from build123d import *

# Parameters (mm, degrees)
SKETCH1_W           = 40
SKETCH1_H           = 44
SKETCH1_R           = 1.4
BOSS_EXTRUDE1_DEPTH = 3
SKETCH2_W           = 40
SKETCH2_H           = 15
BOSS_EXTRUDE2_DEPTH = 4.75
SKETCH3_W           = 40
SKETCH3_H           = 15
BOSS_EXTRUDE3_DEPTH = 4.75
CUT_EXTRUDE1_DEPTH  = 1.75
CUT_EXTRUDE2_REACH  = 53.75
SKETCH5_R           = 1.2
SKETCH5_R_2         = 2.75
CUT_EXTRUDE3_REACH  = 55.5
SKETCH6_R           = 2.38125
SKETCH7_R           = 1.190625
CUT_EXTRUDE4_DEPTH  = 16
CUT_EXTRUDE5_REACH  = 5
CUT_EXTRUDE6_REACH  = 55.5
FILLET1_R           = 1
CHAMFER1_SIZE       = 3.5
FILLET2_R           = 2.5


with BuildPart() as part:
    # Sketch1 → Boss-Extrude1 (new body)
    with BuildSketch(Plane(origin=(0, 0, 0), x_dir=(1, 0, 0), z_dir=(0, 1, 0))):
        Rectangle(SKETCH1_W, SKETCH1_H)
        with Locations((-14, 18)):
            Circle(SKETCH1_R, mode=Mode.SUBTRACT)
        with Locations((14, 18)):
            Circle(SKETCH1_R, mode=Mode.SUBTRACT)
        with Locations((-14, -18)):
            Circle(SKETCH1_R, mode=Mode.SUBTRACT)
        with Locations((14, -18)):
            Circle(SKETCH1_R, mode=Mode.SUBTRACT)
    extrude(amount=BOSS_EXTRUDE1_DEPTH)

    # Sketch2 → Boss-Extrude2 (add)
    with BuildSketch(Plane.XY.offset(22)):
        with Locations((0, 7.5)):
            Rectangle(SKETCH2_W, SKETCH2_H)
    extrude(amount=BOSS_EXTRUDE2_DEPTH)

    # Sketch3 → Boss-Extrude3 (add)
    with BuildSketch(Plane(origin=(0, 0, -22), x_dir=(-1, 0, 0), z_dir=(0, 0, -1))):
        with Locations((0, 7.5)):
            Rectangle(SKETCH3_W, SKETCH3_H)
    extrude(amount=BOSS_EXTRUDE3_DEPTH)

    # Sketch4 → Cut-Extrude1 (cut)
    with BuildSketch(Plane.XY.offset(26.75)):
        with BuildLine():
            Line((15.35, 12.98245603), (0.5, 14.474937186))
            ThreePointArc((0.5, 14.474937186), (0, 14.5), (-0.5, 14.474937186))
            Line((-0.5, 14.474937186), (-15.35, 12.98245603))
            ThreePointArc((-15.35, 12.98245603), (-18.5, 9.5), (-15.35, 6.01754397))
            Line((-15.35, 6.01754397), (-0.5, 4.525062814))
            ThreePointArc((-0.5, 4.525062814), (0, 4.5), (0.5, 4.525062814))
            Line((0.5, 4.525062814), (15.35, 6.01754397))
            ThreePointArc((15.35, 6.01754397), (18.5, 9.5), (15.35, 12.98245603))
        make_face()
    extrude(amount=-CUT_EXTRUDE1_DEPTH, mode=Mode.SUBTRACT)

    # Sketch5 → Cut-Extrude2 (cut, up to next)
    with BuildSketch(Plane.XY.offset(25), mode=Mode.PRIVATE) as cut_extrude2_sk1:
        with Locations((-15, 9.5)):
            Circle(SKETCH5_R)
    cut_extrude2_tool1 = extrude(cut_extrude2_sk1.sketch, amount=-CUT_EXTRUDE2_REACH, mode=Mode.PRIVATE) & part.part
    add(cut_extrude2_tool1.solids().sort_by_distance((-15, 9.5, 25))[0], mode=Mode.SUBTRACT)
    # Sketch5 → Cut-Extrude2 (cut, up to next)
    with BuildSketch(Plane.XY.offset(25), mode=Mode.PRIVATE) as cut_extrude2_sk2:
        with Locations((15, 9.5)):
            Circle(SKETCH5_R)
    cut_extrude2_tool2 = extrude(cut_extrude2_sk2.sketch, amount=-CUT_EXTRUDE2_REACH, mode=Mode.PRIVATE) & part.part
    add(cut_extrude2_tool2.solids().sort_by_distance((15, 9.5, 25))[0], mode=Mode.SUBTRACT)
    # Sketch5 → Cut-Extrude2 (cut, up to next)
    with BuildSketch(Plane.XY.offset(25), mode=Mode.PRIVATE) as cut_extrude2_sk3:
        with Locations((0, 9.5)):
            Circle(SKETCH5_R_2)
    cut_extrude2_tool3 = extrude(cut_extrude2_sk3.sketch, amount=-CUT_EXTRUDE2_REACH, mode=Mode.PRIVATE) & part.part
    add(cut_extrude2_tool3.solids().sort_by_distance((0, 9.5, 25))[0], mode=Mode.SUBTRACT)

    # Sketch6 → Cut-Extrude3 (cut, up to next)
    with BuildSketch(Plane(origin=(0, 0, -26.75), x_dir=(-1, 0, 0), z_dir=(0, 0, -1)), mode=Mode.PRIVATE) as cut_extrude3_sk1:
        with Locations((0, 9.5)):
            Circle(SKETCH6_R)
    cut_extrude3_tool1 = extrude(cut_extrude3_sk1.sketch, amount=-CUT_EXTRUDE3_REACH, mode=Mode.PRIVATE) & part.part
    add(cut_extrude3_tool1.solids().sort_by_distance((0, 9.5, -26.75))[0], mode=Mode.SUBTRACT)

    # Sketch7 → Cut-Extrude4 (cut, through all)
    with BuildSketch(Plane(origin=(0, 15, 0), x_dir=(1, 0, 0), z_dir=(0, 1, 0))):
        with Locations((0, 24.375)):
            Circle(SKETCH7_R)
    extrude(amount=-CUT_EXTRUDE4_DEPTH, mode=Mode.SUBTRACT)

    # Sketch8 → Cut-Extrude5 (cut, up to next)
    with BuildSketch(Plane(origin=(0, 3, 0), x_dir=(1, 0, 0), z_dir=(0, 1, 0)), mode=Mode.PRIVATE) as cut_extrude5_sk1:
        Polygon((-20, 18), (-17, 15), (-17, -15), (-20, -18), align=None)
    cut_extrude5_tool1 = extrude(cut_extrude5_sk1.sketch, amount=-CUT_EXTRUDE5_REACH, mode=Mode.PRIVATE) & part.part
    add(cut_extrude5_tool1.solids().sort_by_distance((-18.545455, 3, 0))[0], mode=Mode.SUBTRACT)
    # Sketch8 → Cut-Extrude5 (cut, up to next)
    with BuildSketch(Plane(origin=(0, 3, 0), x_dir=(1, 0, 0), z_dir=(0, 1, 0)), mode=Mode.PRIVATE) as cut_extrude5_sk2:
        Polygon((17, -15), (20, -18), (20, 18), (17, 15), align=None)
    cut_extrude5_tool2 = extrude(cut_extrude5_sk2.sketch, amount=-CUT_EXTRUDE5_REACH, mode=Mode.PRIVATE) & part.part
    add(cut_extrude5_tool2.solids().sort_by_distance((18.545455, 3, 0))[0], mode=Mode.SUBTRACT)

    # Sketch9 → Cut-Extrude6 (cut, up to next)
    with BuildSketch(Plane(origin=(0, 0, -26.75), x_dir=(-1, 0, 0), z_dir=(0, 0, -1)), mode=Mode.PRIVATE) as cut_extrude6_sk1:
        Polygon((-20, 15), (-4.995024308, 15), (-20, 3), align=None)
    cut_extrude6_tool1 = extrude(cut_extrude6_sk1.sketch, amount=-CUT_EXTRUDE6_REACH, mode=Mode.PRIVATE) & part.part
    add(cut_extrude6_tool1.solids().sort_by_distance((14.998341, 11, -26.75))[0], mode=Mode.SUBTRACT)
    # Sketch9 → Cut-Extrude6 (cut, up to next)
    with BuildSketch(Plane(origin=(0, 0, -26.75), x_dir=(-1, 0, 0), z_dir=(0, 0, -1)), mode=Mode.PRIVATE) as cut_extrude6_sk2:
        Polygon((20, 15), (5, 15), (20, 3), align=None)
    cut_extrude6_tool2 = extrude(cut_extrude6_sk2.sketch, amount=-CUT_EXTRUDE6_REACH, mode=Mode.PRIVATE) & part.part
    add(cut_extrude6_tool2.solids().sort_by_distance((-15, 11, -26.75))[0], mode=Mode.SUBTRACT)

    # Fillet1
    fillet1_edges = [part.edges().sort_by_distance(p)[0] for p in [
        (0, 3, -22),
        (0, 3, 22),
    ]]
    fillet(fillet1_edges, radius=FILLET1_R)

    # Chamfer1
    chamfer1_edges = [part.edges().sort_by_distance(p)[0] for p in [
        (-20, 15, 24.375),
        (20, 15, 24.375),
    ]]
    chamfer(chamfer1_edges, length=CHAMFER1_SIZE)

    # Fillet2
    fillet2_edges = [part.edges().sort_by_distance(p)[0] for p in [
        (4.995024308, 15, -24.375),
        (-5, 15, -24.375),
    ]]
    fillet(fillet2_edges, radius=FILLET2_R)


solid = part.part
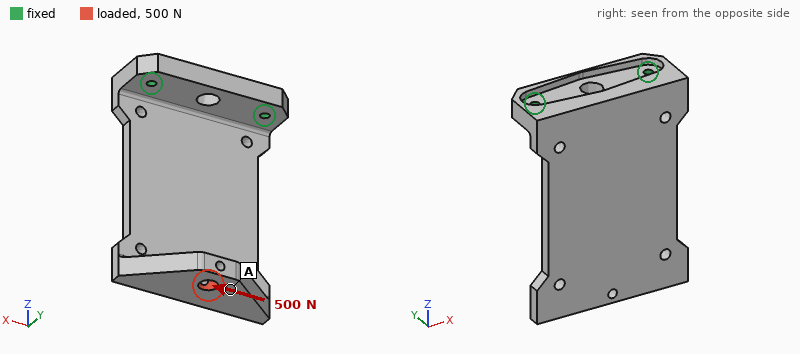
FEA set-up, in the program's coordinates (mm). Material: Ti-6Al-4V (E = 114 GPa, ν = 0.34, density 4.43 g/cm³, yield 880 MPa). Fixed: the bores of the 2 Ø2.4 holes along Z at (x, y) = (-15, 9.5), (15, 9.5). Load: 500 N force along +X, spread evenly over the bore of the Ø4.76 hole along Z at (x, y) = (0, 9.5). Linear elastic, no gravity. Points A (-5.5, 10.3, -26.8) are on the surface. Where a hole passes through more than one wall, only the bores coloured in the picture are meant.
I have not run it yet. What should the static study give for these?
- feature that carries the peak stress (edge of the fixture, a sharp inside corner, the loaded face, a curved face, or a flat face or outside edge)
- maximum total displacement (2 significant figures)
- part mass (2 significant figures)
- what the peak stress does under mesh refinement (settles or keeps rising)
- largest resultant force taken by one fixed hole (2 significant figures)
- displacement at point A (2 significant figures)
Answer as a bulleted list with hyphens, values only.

- edge of the fixture
- 0.29 mm
- 38 g
- keeps rising
- 800 N
- 0.24 mm
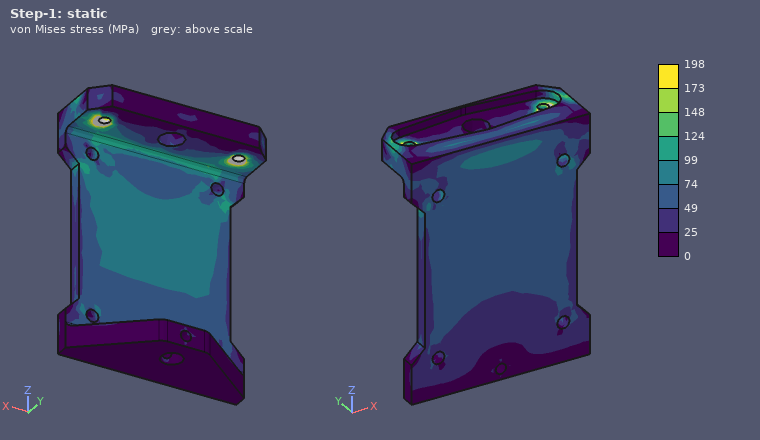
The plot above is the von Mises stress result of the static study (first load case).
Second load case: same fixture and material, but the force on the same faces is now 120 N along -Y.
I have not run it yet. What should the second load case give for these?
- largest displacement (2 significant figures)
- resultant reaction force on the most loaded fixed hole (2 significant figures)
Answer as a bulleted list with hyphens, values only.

- 0.72 mm
- 61 N
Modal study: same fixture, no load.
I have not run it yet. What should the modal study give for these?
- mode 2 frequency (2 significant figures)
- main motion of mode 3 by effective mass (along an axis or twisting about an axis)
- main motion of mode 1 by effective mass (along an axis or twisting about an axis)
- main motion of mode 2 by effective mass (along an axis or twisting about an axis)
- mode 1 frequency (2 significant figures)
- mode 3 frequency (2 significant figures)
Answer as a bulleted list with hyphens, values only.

- 2100 Hz
- along X
- along Y
- along X
- 600 Hz
- 3400 Hz
